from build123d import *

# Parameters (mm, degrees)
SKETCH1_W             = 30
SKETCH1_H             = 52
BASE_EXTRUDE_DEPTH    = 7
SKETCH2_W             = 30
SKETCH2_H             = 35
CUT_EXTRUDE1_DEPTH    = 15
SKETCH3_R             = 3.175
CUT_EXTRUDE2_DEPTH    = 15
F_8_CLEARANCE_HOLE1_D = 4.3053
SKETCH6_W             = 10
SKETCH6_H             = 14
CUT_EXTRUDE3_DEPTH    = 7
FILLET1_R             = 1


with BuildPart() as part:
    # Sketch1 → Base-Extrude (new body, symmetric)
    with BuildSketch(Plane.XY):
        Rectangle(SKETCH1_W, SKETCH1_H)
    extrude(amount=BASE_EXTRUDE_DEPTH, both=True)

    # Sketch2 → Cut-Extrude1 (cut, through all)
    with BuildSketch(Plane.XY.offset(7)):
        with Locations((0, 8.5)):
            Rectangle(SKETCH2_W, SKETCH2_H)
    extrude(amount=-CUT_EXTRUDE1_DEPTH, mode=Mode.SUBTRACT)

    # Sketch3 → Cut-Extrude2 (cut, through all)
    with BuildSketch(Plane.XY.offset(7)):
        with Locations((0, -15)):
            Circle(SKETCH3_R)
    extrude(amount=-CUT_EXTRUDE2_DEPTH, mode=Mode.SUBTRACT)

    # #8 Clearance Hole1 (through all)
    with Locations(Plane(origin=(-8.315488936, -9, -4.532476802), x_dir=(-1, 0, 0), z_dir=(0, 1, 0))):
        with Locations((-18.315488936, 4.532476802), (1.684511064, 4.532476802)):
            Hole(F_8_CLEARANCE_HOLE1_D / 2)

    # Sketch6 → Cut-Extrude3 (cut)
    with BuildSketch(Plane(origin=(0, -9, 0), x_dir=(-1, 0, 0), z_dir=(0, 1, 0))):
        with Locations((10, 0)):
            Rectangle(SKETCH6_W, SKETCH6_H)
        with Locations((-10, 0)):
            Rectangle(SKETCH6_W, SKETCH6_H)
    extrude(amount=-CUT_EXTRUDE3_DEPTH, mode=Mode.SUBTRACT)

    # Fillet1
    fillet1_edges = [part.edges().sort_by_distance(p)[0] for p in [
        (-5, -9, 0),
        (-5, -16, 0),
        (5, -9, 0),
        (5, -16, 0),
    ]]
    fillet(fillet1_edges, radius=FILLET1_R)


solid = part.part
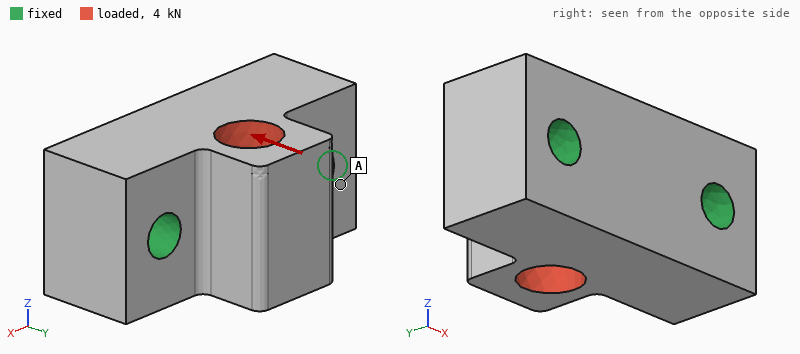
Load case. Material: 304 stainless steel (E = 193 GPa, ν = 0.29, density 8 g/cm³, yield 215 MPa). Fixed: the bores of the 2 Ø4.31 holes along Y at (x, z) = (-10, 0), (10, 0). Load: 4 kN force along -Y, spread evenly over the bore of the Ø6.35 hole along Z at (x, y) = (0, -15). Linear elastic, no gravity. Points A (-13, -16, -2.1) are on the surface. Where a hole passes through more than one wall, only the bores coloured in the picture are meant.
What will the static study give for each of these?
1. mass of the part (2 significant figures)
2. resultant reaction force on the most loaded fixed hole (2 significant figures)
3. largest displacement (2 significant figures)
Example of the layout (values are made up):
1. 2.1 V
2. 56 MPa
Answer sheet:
1. 36 g
2. 2.0 kN
3. 2.9 µm
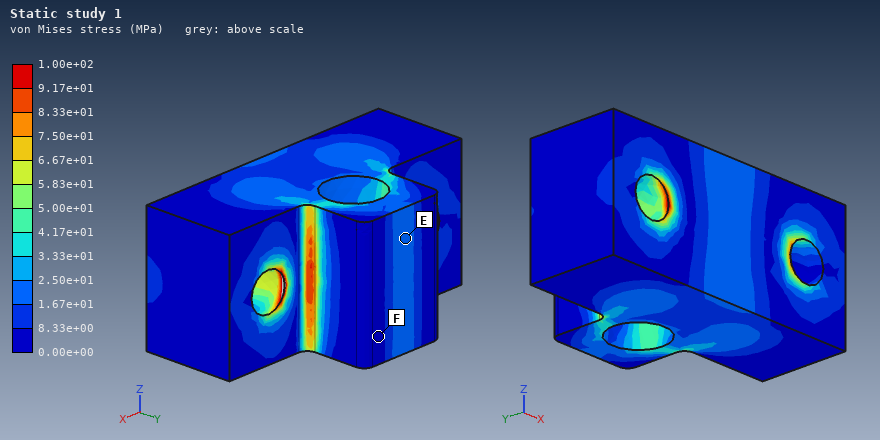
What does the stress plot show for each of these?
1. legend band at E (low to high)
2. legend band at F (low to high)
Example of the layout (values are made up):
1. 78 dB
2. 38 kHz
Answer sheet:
1. 1.67e+01 to 2.50e+01 MPa
2. 0.00e+00 to 8.33e+00 MPa
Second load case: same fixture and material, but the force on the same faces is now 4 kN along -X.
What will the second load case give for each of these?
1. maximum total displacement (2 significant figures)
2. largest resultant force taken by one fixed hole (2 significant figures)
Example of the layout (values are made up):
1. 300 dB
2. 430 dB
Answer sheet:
1. 6.4 µm
2. 2.2 kN
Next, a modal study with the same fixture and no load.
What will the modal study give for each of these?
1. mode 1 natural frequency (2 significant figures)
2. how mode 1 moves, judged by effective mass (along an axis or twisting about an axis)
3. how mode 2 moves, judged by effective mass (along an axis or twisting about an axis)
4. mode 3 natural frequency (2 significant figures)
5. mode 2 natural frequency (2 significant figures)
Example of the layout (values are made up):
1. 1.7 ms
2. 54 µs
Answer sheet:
1. 35 kHz
2. along Z
3. along X
4. 53 kHz
5. 41 kHz
